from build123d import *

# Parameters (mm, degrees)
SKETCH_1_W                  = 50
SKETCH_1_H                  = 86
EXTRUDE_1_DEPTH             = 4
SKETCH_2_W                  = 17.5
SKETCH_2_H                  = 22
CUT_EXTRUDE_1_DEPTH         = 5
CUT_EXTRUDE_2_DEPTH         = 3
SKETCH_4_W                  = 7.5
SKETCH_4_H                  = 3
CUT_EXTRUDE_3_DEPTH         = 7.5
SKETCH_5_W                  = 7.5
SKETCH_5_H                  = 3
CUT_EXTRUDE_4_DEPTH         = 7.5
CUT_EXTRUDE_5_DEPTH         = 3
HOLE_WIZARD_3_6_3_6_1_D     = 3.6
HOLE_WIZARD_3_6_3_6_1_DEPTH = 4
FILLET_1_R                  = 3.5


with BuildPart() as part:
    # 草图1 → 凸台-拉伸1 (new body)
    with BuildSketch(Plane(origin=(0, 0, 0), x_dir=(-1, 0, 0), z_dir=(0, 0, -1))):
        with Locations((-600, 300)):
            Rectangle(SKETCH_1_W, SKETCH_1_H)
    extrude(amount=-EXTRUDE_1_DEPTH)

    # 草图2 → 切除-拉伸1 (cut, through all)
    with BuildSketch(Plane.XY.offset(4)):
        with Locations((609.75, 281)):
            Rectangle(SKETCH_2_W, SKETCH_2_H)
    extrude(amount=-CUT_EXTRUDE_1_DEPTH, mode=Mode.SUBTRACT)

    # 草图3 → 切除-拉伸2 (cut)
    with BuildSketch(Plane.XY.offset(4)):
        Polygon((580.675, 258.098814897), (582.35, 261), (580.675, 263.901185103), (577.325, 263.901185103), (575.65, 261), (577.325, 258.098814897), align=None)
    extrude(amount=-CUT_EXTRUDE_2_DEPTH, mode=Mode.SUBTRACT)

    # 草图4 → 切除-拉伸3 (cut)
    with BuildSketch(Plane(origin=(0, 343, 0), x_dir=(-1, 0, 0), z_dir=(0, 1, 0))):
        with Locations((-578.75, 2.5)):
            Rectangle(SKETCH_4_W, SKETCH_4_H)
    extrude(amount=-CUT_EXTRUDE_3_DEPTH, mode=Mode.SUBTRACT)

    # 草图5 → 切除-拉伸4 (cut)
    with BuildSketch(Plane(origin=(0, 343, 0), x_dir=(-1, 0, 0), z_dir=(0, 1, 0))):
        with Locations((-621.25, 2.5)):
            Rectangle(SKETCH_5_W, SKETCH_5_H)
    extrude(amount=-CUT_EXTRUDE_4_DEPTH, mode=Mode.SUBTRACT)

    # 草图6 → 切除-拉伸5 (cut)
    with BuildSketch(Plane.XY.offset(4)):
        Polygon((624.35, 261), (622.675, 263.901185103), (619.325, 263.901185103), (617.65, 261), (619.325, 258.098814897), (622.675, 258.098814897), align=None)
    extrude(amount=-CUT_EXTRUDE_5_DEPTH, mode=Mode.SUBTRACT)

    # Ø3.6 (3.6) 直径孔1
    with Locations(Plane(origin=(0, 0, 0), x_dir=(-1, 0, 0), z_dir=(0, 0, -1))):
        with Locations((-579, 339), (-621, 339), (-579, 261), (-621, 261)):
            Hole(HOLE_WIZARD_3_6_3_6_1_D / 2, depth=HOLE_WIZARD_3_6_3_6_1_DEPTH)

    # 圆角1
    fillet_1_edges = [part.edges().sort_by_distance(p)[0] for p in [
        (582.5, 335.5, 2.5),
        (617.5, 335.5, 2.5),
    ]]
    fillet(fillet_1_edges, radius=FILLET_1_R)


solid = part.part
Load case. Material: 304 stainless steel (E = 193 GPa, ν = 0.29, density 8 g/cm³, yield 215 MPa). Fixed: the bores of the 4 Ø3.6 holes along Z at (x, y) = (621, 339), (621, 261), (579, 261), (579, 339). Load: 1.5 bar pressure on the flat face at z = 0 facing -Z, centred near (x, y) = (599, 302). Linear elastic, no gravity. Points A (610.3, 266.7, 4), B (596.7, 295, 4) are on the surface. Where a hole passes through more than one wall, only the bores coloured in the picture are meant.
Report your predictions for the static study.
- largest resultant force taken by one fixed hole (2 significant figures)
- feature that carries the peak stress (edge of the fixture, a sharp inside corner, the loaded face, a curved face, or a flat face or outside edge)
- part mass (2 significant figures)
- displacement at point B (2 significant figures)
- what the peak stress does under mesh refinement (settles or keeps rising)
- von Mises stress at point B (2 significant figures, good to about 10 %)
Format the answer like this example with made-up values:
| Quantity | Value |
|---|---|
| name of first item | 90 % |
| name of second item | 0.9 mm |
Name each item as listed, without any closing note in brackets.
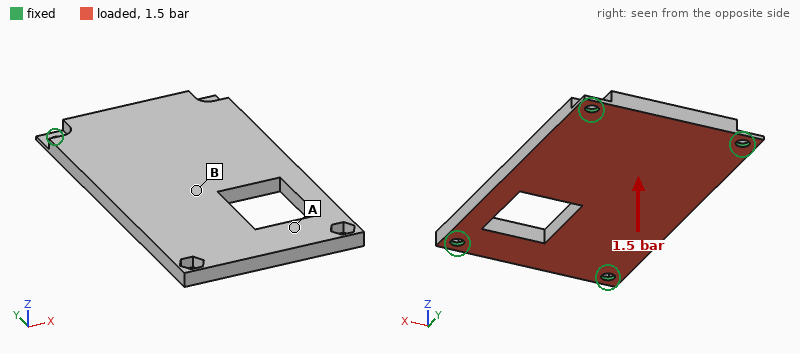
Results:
| Quantity | Value |
|---|---|
| largest resultant force taken by one fixed hole | 470 N |
| feature that carries the peak stress | edge of the fixture |
| part mass | 120 g |
| displacement at point B | 35 µm |
| what the peak stress does under mesh refinement | keeps rising |
| von Mises stress at point B | 28 MPa |
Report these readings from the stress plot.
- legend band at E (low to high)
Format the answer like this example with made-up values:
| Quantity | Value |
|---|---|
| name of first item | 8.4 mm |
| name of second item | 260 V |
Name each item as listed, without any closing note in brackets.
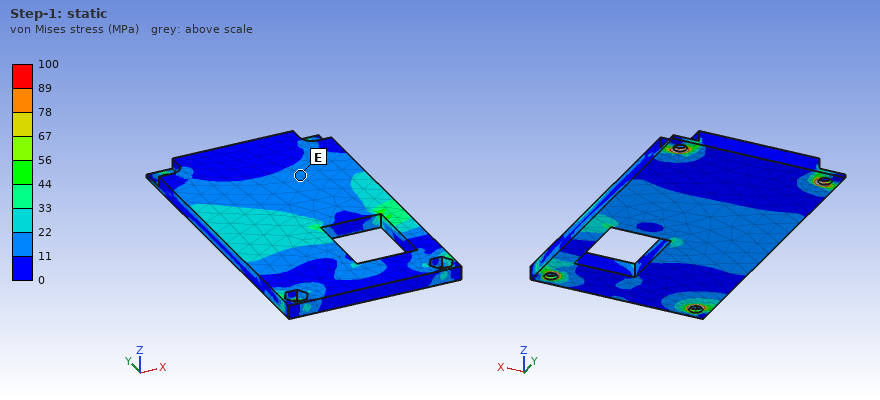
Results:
| Quantity | Value |
|---|---|
| legend band at E | 11 to 22 MPa |
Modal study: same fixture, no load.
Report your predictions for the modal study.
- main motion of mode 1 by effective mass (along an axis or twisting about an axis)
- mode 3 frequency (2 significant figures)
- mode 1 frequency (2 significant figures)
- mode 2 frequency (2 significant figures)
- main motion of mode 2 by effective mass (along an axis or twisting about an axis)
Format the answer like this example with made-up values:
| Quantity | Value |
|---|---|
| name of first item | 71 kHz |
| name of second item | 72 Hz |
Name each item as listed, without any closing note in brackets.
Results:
| Quantity | Value |
|---|---|
| main motion of mode 1 by effective mass | along Z |
| mode 3 frequency | 5800 Hz |
| mode 1 frequency | 2100 Hz |
| mode 2 frequency | 3800 Hz |
| main motion of mode 2 by effective mass | twisting about Y |
